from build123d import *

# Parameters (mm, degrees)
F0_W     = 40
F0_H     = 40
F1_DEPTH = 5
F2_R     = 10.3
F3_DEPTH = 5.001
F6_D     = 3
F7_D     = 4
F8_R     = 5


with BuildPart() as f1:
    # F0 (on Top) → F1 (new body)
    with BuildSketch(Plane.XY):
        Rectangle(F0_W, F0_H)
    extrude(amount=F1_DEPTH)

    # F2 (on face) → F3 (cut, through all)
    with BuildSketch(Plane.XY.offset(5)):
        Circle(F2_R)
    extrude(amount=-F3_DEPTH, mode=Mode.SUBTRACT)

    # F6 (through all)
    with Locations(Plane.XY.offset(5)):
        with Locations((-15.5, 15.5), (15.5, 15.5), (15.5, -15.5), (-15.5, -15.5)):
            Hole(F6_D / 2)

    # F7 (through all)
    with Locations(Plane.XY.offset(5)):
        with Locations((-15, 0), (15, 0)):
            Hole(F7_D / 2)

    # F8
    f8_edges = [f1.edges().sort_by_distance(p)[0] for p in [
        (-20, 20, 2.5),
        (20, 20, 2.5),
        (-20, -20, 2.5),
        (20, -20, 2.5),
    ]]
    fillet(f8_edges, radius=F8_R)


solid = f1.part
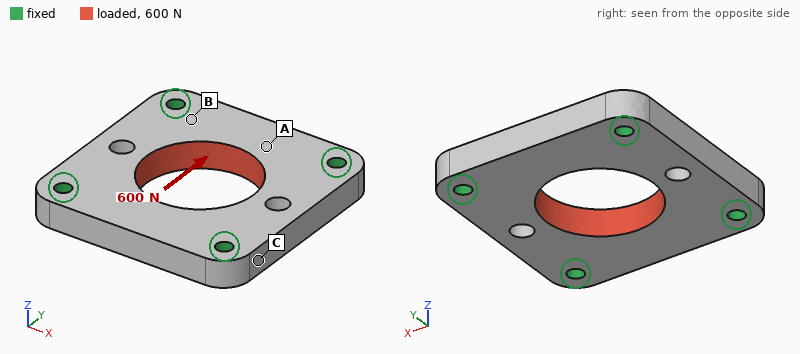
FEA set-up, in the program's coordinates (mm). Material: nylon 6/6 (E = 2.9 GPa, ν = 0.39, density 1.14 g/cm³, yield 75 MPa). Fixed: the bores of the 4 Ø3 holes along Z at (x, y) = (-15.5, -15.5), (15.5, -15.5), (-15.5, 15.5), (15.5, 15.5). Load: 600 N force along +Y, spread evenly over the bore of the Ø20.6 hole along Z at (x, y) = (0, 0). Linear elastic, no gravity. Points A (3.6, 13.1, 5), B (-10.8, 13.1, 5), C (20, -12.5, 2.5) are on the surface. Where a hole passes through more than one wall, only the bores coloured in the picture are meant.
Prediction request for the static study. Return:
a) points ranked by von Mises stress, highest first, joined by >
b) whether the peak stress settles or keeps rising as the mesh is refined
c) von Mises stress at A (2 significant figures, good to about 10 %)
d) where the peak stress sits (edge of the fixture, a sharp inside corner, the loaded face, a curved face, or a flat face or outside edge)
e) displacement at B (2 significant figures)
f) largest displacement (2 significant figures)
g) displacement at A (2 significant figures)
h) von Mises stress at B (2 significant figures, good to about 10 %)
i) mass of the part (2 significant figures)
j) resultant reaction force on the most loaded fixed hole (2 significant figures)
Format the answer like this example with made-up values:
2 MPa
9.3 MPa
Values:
B > A > C
keeps rising
2.2 MPa
edge of the fixture
12 µm
32 µm
28 µm
3.1 MPa
6.8 g
160 N
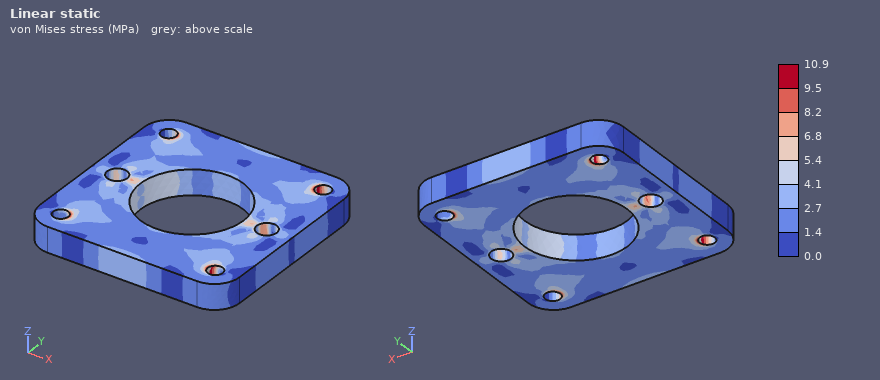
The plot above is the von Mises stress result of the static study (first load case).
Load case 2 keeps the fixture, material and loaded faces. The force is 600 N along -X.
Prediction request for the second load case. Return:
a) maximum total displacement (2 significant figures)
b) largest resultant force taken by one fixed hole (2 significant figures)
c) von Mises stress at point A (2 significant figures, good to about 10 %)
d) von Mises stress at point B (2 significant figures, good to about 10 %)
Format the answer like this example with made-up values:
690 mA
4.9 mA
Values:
32 µm
160 N
3.0 MPa
3.1 MPa
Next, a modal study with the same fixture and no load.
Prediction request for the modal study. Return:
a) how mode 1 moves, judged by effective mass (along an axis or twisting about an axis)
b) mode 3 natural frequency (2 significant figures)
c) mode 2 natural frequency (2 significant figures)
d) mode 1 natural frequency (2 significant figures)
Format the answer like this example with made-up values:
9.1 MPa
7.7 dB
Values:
along Z
7800 Hz
7800 Hz
6700 Hz
